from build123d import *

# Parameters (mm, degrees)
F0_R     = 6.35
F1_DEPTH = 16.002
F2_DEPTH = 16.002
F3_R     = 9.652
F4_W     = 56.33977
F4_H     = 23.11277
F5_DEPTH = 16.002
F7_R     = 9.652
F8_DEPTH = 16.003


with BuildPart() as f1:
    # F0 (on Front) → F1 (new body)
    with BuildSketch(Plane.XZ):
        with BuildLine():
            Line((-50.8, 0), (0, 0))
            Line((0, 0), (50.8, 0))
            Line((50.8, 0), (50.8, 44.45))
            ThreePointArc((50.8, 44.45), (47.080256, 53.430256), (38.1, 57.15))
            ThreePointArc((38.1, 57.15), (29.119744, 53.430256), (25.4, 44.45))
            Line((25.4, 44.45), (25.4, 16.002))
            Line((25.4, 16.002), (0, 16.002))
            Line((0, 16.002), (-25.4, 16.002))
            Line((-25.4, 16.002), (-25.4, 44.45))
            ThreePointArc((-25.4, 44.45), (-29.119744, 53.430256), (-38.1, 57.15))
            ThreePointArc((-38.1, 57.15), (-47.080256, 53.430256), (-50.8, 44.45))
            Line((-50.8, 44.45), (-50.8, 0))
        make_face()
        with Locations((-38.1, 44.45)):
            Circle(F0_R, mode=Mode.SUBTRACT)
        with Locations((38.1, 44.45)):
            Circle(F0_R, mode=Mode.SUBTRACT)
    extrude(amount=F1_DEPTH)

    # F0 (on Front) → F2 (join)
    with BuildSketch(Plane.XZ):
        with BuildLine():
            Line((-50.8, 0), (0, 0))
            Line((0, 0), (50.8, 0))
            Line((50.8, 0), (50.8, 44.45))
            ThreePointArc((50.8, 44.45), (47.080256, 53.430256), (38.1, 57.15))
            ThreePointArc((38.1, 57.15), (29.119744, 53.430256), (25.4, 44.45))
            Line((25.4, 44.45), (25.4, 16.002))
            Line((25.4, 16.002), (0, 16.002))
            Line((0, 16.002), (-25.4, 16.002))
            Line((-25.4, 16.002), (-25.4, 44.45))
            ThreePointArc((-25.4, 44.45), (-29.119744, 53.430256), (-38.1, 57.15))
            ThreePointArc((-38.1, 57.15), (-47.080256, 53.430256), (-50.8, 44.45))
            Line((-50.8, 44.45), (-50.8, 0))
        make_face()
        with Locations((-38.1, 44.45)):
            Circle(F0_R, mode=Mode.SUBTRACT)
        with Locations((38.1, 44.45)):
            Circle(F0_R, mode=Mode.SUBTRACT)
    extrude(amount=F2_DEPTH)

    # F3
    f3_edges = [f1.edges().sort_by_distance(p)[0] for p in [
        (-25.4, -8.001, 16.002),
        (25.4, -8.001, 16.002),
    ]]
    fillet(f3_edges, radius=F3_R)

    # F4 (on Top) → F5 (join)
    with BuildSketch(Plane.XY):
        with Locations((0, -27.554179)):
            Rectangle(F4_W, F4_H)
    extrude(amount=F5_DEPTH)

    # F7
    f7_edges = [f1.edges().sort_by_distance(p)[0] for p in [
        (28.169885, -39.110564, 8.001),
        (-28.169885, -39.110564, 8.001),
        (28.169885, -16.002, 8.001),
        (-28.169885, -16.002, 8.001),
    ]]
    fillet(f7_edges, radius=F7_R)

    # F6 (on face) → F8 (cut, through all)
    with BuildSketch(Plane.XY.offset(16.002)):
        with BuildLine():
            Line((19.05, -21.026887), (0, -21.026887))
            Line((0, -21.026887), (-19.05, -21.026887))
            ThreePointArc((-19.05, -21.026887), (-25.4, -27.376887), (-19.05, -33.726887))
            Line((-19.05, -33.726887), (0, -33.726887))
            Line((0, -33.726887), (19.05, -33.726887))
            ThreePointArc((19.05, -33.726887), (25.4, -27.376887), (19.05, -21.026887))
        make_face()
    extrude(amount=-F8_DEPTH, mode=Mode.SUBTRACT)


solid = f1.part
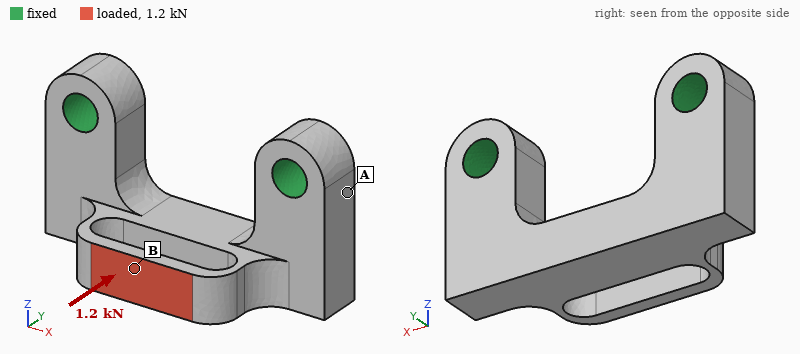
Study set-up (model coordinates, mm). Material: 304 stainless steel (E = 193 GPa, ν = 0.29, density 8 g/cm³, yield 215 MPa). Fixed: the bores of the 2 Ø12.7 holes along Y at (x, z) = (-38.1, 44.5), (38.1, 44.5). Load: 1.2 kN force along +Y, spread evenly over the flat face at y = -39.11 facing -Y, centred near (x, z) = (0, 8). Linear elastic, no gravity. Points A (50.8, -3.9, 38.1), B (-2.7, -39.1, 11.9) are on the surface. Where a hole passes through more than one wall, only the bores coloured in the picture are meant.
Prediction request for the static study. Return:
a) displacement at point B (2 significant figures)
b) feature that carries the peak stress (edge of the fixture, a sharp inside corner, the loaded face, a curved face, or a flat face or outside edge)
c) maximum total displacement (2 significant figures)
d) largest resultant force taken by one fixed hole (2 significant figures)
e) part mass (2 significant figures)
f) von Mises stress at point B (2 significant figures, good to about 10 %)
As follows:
31 µm
a curved face
35 µm
600 N
520 g
65 MPa
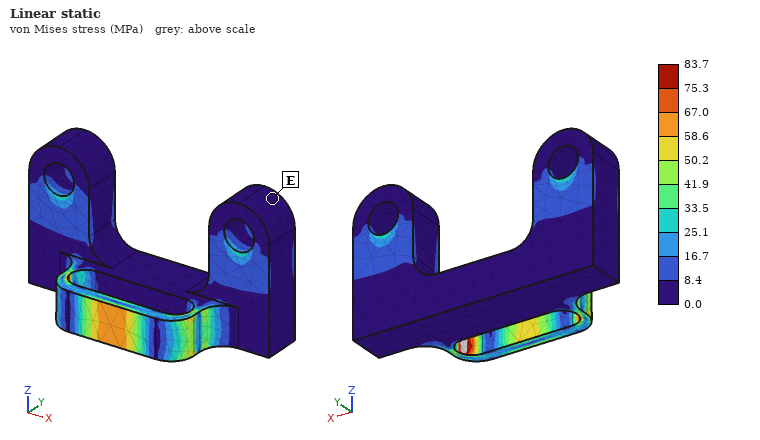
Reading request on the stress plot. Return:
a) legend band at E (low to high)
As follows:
0.0 to 8.4 MPa
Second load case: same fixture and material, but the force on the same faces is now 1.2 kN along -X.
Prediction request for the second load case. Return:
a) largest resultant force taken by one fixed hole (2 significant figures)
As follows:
780 N
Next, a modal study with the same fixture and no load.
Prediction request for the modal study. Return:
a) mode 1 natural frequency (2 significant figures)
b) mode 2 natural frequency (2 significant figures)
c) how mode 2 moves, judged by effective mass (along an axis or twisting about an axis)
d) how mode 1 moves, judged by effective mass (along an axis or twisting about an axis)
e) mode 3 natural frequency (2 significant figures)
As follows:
3700 Hz
5700 Hz
along X
along Y
6900 Hz
